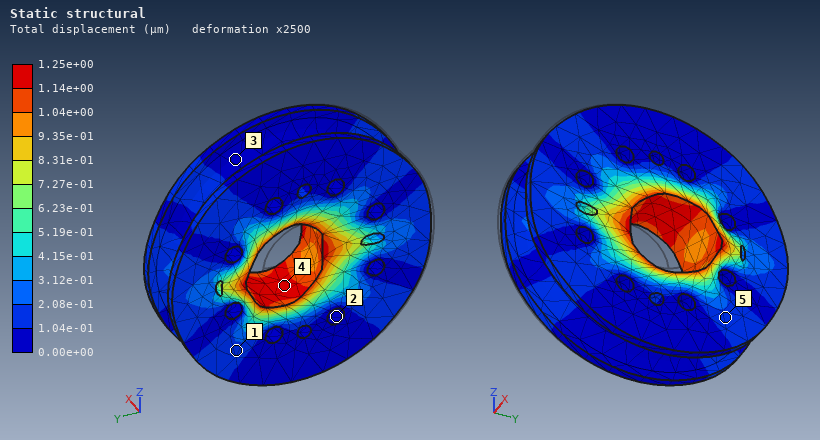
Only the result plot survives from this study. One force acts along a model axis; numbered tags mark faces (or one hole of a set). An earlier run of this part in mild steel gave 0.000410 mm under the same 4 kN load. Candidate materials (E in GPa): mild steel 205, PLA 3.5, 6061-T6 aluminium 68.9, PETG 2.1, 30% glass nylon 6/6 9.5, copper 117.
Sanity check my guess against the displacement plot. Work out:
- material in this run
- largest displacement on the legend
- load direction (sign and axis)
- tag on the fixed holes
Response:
6061-T6 aluminium
1.25e+00 µm
+Y
2
